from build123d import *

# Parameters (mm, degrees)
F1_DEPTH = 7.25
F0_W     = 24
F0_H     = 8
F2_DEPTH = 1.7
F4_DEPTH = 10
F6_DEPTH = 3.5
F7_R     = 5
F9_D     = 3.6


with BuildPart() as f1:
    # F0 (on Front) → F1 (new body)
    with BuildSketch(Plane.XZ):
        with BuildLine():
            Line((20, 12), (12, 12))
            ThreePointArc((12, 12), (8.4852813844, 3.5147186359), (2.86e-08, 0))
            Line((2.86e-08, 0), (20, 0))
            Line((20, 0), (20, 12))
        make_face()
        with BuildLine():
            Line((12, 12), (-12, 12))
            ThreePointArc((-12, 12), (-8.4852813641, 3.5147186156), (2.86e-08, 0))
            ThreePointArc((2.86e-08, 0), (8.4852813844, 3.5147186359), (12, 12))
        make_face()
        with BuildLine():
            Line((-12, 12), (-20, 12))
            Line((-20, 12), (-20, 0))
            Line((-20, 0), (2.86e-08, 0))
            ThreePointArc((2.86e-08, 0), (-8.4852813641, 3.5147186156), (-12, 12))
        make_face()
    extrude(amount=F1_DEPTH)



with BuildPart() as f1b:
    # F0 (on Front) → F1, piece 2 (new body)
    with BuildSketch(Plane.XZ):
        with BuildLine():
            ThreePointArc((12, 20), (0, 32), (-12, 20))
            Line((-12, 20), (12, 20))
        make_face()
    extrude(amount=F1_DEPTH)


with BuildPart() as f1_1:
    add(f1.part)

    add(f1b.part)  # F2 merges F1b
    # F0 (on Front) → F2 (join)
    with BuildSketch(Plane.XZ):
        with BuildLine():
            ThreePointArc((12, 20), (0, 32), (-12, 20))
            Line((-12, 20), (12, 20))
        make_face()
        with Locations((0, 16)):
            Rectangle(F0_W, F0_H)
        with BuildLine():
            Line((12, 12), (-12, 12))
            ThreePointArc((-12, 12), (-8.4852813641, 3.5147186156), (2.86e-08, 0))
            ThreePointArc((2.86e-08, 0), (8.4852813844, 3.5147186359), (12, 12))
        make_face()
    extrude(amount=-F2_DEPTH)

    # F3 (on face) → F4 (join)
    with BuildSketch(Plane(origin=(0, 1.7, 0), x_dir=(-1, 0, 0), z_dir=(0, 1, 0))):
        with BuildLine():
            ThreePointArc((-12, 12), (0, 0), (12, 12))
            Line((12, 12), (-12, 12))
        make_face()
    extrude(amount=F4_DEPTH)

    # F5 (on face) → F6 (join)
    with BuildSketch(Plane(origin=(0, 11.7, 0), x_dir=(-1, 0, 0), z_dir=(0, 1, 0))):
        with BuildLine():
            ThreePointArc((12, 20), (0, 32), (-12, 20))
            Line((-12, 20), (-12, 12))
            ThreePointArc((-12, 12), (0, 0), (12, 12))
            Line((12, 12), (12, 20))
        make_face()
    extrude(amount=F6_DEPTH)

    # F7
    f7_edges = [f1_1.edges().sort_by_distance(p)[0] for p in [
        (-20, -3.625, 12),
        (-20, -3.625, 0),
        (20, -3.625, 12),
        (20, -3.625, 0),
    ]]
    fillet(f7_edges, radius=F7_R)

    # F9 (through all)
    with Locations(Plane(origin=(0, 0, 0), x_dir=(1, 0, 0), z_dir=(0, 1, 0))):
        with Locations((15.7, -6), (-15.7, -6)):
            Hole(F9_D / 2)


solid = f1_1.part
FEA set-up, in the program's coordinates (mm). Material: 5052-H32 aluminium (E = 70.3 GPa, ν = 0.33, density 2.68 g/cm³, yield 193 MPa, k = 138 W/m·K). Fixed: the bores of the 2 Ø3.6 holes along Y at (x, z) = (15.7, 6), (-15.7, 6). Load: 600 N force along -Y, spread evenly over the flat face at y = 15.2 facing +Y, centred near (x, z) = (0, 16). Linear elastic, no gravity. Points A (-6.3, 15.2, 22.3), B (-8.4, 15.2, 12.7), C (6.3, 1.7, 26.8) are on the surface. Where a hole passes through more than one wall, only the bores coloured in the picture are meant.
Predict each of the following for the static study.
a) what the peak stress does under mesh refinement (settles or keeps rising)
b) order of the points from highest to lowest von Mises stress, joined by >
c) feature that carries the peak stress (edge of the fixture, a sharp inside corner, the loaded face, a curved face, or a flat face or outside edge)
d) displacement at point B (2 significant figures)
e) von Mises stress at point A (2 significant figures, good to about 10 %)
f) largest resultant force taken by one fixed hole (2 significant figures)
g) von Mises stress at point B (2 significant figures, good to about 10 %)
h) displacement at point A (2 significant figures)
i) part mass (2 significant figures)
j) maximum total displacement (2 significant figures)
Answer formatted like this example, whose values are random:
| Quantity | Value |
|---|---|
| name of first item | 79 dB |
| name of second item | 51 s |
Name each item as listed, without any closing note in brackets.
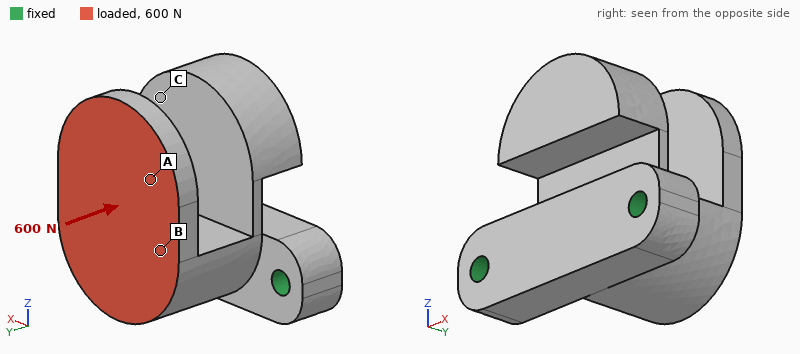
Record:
| Quantity | Value |
|---|---|
| what the peak stress does under mesh refinement | keeps rising |
| order of the points from highest to lowest von Mises stress, joined by > | B > A > C |
| feature that carries the peak stress | edge of the fixture |
| displacement at point B | 0.026 mm |
| von Mises stress at point A | 15 MPa |
| largest resultant force taken by one fixed hole | 320 N |
| von Mises stress at point B | 54 MPa |
| displacement at point A | 0.061 mm |
| part mass | 28 g |
| maximum total displacement | 0.11 mm |
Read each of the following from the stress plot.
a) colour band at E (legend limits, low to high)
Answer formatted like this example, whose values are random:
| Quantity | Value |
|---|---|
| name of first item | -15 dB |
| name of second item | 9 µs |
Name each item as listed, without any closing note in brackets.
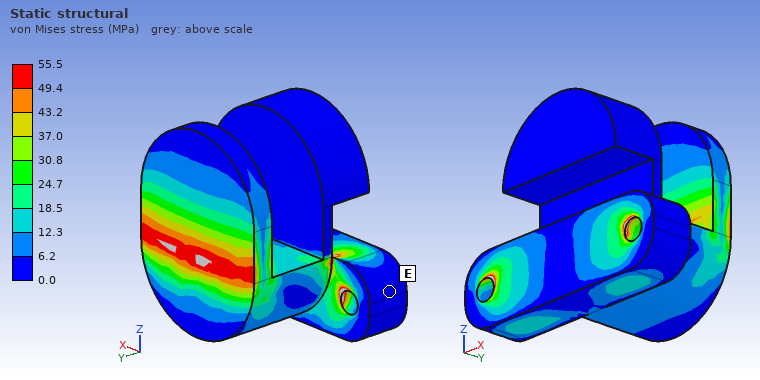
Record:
| Quantity | Value |
|---|---|
| colour band at E | 0.0 to 6.2 MPa |
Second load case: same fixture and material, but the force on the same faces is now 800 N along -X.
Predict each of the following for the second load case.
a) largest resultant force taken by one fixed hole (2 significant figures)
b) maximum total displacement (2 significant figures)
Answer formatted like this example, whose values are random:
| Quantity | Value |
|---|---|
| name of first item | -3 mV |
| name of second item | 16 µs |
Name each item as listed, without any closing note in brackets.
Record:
| Quantity | Value |
|---|---|
| largest resultant force taken by one fixed hole | 740 N |
| maximum total displacement | 31 µm |
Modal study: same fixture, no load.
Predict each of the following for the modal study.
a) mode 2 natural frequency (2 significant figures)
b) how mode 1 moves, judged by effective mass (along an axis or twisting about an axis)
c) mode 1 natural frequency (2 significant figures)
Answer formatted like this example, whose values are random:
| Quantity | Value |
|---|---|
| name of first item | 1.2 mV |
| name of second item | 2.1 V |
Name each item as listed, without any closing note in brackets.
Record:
| Quantity | Value |
|---|---|
| mode 2 natural frequency | 5300 Hz |
| how mode 1 moves, judged by effective mass | along Y |
| mode 1 natural frequency | 1800 Hz |
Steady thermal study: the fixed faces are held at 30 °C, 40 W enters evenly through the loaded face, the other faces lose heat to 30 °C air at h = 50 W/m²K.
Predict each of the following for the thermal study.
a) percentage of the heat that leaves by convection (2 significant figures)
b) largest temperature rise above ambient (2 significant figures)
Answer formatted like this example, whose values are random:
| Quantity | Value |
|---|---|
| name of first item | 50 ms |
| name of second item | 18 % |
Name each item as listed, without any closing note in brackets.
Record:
| Quantity | Value |
|---|---|
| percentage of the heat that leaves by convection | 9.3 % |
| largest temperature rise above ambient | 55 K |
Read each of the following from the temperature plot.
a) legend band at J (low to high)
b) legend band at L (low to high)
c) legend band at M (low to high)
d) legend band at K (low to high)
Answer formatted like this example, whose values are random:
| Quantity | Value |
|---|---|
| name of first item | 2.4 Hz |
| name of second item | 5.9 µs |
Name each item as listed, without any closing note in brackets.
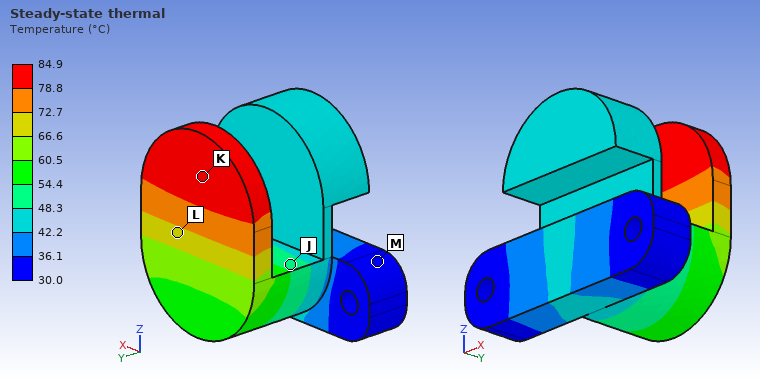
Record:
| Quantity | Value |
|---|---|
| legend band at J | 48.3 to 54.4 °C |
| legend band at L | 66.6 to 72.7 °C |
| legend band at M | 30.0 to 36.1 °C |
| legend band at K | 78.8 to 84.9 °C |
